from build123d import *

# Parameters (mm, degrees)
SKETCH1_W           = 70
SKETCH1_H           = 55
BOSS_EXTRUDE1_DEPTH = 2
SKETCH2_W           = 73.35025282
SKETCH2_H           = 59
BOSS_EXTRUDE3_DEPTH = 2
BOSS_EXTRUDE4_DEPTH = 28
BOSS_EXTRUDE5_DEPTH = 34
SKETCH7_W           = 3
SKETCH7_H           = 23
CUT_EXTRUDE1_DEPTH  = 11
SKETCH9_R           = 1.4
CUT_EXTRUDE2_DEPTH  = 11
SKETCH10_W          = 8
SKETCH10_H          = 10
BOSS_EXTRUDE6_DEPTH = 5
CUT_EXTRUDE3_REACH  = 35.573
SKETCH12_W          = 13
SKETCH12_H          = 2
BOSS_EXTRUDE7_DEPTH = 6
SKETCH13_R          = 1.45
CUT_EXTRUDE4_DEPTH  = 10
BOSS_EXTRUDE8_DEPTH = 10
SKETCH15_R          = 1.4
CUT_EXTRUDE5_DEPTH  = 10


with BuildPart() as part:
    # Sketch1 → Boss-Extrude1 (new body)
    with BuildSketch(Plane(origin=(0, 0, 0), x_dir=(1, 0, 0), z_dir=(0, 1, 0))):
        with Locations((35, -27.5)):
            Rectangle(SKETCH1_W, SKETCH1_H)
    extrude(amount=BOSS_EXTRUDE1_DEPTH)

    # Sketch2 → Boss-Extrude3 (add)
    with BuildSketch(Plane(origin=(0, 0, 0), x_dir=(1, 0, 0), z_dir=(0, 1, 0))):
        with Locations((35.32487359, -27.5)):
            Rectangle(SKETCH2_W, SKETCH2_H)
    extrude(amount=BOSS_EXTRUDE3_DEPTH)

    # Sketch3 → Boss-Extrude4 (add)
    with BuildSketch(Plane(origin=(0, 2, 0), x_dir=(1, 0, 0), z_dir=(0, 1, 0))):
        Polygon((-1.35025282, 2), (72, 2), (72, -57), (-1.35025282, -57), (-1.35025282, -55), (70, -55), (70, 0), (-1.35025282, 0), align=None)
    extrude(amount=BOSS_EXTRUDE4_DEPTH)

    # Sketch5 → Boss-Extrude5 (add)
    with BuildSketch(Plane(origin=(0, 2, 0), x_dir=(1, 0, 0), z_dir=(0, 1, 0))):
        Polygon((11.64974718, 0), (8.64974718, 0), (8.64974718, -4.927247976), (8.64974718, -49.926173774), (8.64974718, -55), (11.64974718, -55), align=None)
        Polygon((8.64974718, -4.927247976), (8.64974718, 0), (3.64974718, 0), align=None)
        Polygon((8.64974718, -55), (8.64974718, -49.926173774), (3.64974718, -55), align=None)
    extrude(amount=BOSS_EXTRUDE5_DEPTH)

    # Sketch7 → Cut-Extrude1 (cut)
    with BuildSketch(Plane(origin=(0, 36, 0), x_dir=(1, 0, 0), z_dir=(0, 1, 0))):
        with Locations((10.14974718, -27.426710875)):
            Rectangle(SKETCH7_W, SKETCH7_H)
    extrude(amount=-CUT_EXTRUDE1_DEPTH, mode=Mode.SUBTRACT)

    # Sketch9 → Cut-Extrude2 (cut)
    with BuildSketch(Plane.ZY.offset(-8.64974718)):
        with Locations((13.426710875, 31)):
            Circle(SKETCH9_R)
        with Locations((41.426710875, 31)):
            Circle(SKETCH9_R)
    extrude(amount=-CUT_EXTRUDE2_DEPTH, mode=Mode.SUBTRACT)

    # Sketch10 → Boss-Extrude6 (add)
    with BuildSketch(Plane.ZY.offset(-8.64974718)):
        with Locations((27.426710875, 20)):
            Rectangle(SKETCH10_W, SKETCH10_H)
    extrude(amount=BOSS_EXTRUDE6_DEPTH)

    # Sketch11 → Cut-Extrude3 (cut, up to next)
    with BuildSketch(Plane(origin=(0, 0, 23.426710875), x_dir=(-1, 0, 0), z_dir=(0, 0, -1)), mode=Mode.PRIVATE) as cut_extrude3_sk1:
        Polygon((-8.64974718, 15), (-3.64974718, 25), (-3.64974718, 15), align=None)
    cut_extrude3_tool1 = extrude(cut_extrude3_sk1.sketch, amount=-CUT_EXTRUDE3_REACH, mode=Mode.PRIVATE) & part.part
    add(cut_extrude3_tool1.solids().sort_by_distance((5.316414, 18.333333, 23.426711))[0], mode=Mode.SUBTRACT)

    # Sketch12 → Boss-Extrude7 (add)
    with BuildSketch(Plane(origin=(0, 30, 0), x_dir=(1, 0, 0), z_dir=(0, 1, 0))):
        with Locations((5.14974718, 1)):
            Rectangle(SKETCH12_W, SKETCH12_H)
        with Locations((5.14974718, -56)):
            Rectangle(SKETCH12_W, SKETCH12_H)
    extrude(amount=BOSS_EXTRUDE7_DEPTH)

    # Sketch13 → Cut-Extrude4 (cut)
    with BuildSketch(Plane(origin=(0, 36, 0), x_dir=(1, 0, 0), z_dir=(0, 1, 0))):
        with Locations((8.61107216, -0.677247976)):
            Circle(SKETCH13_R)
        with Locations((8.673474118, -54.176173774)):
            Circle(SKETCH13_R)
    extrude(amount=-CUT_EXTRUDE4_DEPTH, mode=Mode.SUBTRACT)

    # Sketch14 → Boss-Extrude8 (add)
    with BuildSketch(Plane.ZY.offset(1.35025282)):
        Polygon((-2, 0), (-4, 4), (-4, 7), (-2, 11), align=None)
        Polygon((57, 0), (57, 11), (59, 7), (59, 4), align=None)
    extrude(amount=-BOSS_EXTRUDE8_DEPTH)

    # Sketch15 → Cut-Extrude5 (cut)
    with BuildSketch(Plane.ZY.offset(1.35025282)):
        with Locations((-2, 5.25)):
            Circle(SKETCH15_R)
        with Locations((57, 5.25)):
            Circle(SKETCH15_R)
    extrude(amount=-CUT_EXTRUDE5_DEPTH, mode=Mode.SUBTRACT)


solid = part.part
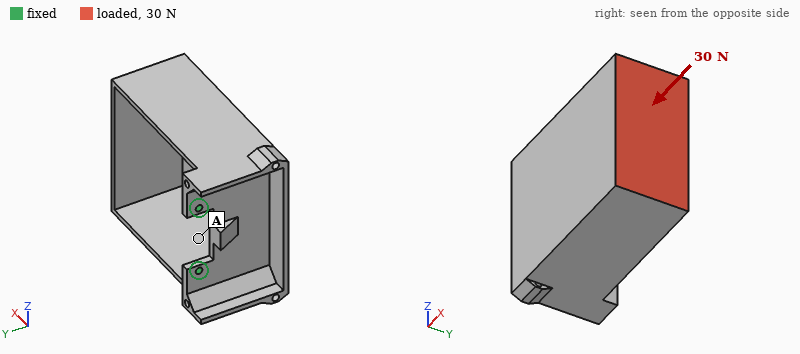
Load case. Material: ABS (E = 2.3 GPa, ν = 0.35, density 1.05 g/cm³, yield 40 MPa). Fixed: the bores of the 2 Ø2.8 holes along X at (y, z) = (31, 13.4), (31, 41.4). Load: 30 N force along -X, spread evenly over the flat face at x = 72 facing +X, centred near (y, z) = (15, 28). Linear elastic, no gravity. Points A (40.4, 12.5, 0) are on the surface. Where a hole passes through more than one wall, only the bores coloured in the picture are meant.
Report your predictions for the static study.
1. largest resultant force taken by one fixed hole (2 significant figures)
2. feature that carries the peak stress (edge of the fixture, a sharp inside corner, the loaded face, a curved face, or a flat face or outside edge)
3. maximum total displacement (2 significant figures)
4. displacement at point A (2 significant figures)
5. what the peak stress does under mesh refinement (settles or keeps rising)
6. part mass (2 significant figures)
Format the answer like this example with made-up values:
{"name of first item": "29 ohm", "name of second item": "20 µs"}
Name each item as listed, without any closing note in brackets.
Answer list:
{"largest resultant force taken by one fixed hole": "15 N", "feature that carries the peak stress": "edge of the fixture", "maximum total displacement": "1.1 mm", "displacement at point A": "0.59 mm", "what the peak stress does under mesh refinement": "keeps rising", "part mass": "27 g"}
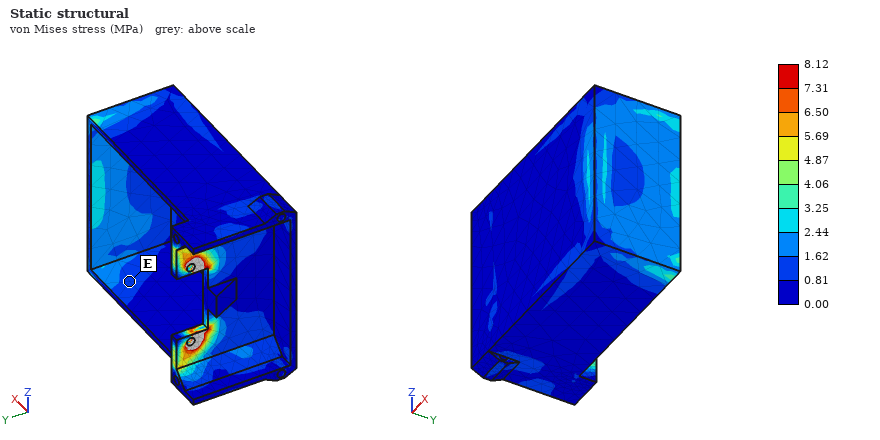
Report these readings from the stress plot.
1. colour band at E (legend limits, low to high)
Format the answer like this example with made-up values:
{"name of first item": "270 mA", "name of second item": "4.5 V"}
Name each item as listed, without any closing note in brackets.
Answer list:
{"colour band at E": "0.81 to 1.62 MPa"}
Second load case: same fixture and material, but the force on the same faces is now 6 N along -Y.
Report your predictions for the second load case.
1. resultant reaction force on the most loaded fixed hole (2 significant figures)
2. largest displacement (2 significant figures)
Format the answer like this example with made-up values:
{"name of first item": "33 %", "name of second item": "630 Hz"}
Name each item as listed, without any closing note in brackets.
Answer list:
{"resultant reaction force on the most loaded fixed hole": "3.1 N", "largest displacement": "1.1 mm"}
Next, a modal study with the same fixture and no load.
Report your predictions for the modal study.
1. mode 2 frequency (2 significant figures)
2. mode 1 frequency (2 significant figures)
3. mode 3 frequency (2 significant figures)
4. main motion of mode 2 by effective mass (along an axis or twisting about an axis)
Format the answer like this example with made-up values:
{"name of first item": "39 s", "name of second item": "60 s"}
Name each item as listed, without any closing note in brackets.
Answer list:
{"mode 2 frequency": "140 Hz", "mode 1 frequency": "120 Hz", "mode 3 frequency": "620 Hz", "main motion of mode 2 by effective mass": "along Z"}
